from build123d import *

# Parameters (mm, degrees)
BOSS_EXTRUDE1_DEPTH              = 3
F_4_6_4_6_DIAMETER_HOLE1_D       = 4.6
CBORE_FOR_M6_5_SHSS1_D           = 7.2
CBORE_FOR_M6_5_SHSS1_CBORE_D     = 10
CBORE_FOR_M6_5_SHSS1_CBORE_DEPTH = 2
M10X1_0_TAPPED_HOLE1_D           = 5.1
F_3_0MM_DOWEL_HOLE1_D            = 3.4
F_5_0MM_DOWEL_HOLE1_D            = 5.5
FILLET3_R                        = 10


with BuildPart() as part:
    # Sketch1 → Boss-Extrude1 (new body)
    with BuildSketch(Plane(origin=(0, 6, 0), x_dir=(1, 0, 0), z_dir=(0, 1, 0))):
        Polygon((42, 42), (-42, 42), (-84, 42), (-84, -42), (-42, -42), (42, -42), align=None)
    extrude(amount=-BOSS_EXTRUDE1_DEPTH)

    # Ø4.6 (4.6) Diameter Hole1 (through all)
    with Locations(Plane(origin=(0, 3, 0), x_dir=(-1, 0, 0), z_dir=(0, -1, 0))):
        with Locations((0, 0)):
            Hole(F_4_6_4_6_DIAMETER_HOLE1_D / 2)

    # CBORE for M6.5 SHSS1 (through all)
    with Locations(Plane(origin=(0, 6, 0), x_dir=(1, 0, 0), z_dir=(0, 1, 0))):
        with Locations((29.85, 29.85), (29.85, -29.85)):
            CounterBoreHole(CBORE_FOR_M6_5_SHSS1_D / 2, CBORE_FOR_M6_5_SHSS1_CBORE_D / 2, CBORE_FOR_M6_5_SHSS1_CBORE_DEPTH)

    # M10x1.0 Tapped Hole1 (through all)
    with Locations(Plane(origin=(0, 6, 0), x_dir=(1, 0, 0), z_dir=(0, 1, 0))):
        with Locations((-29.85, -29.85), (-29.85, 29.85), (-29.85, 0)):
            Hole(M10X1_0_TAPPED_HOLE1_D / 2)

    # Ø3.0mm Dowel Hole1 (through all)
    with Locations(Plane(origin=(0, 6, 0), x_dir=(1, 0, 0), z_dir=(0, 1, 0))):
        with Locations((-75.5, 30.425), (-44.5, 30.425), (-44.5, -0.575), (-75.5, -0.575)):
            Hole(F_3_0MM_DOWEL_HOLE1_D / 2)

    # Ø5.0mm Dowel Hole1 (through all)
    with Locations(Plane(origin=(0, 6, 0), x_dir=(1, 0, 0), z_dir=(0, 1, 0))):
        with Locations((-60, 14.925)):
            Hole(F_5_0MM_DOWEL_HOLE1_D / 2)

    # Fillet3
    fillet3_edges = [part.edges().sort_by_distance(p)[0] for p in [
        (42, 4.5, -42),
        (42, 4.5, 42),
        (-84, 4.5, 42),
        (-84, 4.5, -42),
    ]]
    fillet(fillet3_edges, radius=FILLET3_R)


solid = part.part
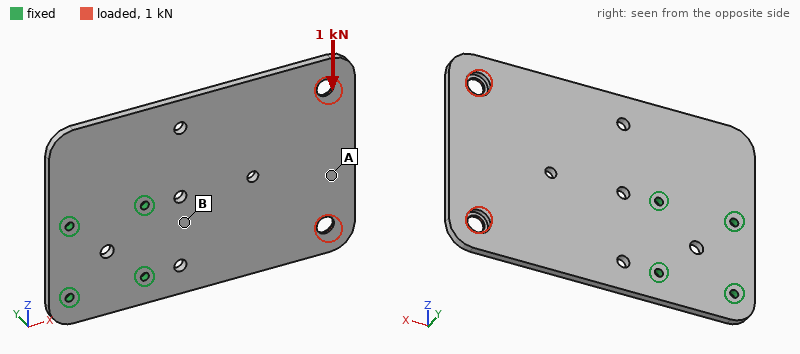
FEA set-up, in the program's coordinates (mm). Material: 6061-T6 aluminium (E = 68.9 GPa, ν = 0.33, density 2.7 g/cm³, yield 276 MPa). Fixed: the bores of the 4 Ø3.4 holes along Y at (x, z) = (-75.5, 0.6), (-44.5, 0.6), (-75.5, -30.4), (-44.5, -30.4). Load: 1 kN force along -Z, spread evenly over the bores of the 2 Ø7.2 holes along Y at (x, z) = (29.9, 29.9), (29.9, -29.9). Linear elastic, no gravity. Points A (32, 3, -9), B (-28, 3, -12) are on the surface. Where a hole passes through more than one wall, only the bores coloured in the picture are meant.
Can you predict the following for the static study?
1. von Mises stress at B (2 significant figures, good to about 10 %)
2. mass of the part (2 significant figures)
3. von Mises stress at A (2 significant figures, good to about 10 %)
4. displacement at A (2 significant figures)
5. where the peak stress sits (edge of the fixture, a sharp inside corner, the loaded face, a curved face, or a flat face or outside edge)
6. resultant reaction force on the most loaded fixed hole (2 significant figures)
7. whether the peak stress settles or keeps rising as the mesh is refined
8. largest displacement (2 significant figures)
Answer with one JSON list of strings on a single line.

["23 MPa", "83 g", "8.9 MPa", "0.058 mm", "edge of the fixture", "1.5 kN", "keeps rising", "0.17 mm"]
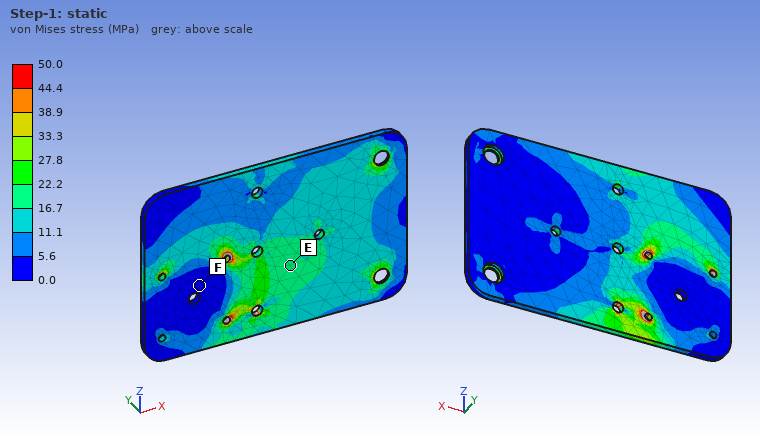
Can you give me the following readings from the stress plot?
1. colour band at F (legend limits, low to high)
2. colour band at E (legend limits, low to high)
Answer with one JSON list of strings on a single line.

["0.0 to 5.6 MPa", "16.7 to 22.2 MPa"]
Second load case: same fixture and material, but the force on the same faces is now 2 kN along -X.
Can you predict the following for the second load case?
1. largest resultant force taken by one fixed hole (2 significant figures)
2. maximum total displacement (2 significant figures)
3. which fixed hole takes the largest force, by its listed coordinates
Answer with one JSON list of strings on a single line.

["1.1 kN", "0.61 mm", "(-44.5, 0.6)"]
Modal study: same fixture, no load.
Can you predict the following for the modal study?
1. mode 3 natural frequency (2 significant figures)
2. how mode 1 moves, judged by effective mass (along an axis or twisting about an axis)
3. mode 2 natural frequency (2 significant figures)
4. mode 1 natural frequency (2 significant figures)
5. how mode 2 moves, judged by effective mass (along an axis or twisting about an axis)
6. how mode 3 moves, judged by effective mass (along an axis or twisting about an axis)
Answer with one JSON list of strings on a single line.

["1500 Hz", "along Y", "720 Hz", "310 Hz", "twisting about X", "along Y"]
